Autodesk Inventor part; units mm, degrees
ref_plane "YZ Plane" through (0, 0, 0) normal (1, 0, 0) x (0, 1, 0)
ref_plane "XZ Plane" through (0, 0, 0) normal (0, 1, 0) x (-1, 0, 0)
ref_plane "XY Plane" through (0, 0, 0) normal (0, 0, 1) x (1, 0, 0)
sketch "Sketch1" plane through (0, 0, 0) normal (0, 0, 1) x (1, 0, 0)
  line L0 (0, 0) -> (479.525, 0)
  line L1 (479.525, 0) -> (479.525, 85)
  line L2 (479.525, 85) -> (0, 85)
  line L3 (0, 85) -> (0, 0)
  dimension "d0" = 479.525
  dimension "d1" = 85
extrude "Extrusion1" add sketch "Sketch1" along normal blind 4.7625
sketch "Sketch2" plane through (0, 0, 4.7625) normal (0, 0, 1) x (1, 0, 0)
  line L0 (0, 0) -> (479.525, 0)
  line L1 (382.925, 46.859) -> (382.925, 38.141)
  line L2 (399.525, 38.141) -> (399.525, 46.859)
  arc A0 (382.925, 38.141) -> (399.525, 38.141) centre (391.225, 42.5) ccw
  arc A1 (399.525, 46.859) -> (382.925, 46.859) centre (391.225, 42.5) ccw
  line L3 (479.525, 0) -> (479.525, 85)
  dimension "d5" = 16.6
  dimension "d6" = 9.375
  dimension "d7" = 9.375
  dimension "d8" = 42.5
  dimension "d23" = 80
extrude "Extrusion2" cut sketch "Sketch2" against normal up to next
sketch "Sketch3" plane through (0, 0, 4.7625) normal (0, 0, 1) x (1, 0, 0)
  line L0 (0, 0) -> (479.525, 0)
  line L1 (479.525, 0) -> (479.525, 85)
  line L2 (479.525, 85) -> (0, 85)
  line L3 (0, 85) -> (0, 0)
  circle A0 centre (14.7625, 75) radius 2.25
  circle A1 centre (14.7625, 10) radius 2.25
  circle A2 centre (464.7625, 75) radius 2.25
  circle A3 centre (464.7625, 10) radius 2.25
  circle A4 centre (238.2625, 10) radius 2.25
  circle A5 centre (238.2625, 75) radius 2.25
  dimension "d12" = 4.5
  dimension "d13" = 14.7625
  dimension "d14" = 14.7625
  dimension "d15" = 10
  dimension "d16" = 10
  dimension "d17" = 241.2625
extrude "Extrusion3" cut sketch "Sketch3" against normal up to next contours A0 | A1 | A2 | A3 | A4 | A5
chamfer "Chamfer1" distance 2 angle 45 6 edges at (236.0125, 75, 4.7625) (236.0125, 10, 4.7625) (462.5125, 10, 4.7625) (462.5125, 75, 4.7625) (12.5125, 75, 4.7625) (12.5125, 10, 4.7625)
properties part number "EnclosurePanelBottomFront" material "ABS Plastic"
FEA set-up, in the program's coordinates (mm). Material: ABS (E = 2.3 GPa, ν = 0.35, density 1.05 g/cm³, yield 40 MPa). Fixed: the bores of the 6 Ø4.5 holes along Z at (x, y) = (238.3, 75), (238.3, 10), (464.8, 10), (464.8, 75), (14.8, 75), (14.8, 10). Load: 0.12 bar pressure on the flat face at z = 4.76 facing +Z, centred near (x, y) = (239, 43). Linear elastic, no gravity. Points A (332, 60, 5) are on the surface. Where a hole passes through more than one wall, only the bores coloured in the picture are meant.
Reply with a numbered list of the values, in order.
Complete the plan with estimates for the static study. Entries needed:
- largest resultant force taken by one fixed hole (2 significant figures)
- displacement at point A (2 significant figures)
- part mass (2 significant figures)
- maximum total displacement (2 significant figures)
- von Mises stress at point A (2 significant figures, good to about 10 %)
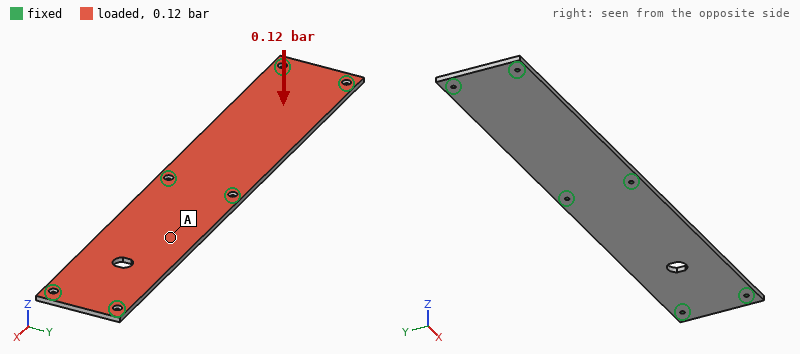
1. 140 N
2. 4.1 mm
3. 200 g
4. 4.7 mm
5. 6.0 MPa
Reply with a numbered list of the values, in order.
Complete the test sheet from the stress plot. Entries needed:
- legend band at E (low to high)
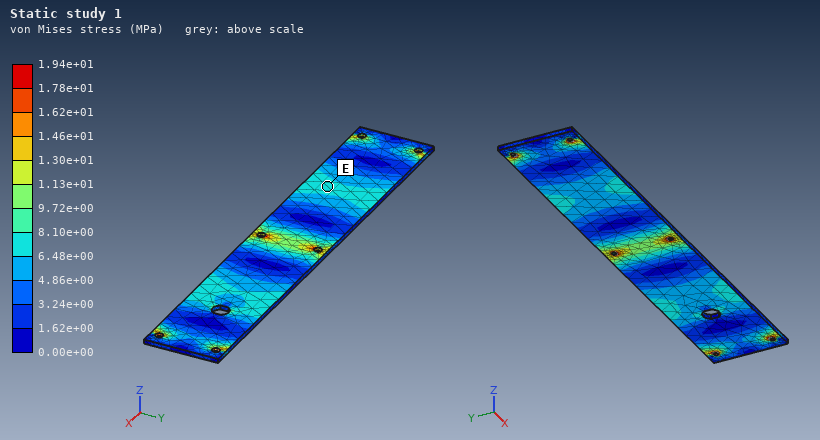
1. 6.48e+00 to 8.10e+00 MPa
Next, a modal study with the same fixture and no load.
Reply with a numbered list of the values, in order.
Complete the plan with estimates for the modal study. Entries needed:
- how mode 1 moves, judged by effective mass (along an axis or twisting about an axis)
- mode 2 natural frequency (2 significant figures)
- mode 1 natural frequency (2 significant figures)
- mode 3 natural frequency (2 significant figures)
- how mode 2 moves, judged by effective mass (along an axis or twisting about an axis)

1. twisting about Y
2. 130 Hz
3. 120 Hz
4. 270 Hz
5. along Z
